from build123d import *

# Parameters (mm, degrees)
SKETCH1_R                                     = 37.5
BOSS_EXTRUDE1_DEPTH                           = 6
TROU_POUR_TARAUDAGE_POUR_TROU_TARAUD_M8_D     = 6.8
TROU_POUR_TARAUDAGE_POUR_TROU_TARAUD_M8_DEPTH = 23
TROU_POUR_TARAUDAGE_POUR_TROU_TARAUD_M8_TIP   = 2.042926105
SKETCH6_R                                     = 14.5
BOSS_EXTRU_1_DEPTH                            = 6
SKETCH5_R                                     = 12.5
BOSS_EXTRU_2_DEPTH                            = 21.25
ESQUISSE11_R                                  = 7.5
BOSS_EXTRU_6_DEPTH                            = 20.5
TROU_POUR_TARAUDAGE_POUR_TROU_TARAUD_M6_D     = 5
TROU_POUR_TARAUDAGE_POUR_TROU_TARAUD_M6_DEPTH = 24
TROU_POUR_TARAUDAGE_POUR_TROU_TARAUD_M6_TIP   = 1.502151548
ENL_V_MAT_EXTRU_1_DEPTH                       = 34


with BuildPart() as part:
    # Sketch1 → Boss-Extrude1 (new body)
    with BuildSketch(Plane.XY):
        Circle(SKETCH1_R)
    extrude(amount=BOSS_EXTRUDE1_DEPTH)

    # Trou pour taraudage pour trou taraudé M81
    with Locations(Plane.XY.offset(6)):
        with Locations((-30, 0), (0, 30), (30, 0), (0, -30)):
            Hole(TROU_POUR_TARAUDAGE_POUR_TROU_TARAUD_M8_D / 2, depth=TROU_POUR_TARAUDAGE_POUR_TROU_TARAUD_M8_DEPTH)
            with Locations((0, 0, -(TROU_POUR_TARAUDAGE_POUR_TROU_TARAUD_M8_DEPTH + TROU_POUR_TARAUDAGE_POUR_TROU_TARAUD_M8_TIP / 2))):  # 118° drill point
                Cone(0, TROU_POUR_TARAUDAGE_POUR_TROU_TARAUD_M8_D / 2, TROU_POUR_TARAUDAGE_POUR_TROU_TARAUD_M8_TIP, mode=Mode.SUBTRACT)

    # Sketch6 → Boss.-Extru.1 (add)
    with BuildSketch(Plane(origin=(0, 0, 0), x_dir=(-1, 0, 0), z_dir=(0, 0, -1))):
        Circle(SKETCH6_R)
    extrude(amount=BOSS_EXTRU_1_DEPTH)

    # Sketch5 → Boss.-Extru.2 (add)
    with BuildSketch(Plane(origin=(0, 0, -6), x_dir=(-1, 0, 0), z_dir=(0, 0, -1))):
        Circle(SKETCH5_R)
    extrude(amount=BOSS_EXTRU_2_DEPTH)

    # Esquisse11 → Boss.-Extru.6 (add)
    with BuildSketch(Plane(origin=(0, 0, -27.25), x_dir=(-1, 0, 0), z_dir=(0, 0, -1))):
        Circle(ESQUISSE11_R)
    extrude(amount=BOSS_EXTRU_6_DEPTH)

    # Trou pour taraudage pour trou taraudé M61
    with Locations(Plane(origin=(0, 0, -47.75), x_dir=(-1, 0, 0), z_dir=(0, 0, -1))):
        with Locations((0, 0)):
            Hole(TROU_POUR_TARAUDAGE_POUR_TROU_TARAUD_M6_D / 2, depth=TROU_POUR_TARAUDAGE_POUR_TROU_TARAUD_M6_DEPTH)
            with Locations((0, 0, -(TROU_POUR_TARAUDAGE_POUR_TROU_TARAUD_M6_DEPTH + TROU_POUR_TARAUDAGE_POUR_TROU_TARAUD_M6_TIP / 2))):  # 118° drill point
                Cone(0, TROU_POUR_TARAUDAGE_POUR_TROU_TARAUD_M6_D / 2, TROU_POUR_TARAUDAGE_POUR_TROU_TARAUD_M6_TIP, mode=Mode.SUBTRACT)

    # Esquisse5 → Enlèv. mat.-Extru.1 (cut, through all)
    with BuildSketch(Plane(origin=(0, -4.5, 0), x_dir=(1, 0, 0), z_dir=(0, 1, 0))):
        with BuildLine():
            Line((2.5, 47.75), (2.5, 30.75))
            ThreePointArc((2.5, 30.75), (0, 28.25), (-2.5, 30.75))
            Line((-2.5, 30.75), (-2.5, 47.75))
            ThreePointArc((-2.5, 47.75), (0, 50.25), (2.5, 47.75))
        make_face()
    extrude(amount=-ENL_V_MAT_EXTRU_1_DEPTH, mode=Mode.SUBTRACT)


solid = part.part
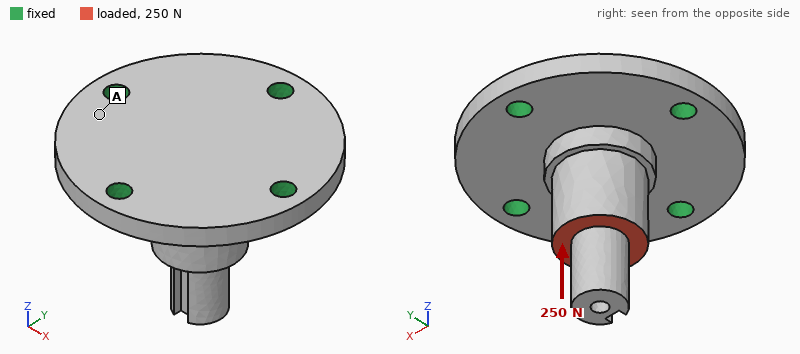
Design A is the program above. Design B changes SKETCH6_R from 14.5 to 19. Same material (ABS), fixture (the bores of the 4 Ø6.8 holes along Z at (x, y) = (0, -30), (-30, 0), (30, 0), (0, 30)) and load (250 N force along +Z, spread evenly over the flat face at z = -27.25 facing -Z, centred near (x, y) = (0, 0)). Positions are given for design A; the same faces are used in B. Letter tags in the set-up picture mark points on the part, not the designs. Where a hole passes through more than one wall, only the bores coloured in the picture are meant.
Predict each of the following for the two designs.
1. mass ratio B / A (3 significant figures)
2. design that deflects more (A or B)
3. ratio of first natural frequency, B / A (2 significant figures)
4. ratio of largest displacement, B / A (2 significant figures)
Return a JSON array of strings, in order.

["1.07", "A", "1.2", "0.68"]
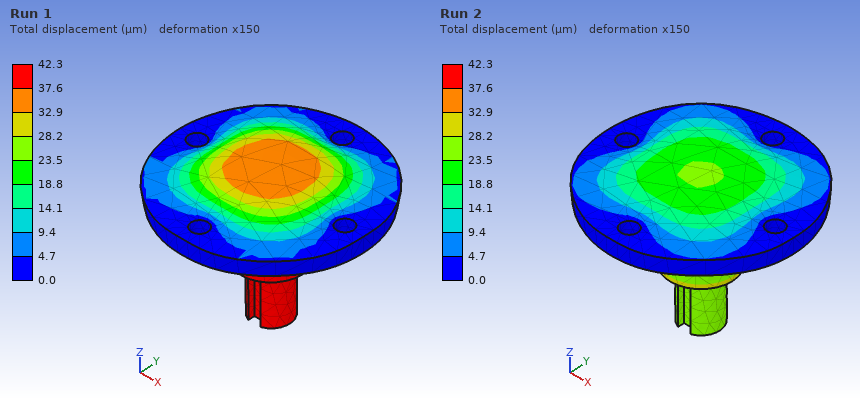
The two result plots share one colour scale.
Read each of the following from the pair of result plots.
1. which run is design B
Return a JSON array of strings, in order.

["Run 2"]
